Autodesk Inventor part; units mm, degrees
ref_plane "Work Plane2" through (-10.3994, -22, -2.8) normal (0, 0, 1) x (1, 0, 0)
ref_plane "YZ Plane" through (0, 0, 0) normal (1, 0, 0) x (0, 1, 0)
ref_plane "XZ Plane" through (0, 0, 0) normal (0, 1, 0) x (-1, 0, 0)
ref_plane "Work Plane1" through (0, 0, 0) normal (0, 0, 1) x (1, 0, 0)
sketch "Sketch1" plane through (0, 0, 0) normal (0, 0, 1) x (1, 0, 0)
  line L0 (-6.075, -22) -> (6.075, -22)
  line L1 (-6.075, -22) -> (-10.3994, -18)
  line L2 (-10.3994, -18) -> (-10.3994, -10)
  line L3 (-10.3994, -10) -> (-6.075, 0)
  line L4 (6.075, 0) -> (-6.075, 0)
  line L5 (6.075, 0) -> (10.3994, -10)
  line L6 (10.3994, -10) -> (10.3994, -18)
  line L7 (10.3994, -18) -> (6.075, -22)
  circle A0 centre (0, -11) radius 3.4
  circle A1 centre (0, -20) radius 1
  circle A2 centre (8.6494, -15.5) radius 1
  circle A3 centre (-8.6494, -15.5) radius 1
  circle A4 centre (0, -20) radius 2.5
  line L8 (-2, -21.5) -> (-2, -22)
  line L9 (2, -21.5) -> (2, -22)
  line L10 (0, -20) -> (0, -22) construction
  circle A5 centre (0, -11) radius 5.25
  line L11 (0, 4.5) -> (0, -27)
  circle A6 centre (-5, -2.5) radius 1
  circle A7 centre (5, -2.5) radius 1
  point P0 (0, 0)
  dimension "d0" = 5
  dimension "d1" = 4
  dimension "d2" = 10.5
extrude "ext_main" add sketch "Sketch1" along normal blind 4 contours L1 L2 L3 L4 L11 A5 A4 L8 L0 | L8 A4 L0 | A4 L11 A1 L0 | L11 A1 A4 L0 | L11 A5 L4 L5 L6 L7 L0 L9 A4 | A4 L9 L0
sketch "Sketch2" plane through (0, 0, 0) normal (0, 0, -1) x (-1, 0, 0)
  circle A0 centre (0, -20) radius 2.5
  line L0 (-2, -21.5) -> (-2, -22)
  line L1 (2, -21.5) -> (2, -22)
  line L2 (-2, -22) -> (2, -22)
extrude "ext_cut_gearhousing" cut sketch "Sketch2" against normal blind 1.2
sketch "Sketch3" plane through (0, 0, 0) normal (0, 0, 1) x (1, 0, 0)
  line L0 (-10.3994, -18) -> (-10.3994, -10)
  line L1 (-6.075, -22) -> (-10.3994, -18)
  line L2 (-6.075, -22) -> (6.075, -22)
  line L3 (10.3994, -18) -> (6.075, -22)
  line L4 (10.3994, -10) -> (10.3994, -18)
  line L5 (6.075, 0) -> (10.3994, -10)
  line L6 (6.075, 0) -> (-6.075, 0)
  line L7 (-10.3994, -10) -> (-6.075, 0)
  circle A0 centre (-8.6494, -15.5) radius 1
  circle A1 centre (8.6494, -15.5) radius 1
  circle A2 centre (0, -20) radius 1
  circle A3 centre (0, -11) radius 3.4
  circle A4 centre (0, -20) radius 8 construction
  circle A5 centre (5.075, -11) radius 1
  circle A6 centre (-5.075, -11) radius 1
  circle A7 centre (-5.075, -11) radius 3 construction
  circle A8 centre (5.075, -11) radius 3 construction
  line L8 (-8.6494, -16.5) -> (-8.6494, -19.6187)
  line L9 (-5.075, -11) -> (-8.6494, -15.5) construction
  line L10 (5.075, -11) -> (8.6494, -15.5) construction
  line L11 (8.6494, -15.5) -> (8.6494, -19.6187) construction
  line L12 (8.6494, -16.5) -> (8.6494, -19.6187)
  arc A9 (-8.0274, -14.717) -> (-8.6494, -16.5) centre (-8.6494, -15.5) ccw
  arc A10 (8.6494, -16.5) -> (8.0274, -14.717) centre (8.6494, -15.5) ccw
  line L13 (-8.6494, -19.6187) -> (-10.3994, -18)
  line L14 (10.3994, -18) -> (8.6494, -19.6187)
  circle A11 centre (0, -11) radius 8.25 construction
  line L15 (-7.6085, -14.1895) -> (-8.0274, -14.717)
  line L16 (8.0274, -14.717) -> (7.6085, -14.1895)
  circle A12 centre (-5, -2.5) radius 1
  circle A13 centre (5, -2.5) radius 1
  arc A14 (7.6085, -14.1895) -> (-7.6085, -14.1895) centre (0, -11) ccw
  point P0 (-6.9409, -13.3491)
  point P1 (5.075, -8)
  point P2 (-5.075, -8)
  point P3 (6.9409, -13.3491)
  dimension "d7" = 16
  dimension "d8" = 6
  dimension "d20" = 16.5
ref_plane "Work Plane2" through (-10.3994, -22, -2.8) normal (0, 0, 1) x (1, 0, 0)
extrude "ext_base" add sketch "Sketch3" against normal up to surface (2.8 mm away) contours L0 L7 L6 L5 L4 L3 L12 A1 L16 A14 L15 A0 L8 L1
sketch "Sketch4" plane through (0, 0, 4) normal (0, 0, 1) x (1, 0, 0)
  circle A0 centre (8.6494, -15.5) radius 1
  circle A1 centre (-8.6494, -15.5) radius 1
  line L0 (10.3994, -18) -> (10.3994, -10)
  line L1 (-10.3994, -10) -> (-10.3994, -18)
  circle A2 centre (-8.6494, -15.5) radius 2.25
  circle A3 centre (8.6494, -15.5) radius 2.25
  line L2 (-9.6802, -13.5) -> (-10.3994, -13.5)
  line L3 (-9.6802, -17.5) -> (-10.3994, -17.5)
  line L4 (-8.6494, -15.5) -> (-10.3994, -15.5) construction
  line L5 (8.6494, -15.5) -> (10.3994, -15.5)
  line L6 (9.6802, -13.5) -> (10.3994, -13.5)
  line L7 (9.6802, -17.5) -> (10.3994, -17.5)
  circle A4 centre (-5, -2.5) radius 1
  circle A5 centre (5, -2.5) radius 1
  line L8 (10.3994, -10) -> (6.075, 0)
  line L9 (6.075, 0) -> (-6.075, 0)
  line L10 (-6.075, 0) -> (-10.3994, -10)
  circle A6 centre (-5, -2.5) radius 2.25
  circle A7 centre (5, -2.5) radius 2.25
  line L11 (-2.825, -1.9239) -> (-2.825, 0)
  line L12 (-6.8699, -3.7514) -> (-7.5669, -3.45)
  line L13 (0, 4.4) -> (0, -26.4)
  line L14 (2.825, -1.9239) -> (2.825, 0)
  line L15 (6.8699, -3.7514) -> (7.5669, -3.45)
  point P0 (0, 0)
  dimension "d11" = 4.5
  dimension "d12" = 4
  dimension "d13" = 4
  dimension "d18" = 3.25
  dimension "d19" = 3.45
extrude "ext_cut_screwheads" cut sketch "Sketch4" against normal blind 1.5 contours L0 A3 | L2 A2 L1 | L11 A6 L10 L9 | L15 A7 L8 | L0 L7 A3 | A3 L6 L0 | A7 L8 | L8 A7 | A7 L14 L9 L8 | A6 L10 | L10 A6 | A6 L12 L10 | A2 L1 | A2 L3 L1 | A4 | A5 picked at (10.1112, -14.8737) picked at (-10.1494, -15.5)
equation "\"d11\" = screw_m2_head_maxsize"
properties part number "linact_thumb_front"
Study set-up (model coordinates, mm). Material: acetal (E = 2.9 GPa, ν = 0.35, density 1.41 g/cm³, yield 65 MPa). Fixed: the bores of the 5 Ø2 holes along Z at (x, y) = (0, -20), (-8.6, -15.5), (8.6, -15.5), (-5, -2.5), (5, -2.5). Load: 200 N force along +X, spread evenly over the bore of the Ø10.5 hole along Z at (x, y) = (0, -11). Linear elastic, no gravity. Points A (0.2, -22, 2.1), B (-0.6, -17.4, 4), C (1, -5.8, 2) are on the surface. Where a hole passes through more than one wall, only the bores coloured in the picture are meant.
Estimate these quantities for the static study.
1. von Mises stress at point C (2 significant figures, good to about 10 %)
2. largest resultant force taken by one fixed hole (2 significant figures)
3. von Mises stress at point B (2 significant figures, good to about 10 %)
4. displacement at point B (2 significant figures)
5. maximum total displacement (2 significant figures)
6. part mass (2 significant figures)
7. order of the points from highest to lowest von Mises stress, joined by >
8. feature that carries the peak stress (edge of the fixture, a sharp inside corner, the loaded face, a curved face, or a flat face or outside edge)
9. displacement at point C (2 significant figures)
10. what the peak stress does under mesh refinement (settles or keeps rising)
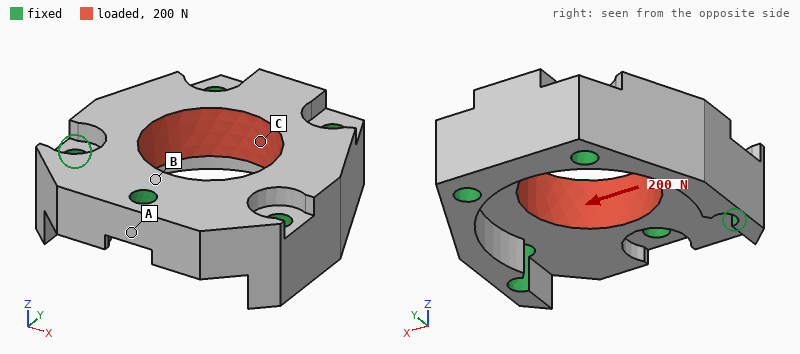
3.5 MPa
43 N
1.4 MPa
2.4 µm
12 µm
1.9 g
C > B > A
edge of the fixture
5.9 µm
keeps rising
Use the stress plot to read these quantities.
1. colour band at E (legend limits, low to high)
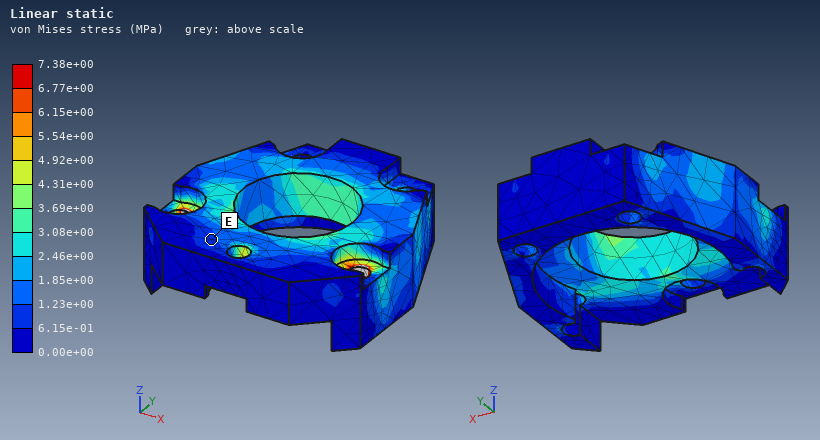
6.15e-01 to 1.23e+00 MPa
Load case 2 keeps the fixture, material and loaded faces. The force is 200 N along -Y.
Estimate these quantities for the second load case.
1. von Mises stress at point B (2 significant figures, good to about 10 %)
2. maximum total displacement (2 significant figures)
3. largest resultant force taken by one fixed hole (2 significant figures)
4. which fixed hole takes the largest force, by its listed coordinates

2.3 MPa
8.2 µm
50 N
(0, -20)
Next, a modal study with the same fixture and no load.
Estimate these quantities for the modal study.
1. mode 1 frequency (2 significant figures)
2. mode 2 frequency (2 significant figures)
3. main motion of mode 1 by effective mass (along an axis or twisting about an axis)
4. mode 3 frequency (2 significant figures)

23 kHz
24 kHz
along Z
25 kHz
